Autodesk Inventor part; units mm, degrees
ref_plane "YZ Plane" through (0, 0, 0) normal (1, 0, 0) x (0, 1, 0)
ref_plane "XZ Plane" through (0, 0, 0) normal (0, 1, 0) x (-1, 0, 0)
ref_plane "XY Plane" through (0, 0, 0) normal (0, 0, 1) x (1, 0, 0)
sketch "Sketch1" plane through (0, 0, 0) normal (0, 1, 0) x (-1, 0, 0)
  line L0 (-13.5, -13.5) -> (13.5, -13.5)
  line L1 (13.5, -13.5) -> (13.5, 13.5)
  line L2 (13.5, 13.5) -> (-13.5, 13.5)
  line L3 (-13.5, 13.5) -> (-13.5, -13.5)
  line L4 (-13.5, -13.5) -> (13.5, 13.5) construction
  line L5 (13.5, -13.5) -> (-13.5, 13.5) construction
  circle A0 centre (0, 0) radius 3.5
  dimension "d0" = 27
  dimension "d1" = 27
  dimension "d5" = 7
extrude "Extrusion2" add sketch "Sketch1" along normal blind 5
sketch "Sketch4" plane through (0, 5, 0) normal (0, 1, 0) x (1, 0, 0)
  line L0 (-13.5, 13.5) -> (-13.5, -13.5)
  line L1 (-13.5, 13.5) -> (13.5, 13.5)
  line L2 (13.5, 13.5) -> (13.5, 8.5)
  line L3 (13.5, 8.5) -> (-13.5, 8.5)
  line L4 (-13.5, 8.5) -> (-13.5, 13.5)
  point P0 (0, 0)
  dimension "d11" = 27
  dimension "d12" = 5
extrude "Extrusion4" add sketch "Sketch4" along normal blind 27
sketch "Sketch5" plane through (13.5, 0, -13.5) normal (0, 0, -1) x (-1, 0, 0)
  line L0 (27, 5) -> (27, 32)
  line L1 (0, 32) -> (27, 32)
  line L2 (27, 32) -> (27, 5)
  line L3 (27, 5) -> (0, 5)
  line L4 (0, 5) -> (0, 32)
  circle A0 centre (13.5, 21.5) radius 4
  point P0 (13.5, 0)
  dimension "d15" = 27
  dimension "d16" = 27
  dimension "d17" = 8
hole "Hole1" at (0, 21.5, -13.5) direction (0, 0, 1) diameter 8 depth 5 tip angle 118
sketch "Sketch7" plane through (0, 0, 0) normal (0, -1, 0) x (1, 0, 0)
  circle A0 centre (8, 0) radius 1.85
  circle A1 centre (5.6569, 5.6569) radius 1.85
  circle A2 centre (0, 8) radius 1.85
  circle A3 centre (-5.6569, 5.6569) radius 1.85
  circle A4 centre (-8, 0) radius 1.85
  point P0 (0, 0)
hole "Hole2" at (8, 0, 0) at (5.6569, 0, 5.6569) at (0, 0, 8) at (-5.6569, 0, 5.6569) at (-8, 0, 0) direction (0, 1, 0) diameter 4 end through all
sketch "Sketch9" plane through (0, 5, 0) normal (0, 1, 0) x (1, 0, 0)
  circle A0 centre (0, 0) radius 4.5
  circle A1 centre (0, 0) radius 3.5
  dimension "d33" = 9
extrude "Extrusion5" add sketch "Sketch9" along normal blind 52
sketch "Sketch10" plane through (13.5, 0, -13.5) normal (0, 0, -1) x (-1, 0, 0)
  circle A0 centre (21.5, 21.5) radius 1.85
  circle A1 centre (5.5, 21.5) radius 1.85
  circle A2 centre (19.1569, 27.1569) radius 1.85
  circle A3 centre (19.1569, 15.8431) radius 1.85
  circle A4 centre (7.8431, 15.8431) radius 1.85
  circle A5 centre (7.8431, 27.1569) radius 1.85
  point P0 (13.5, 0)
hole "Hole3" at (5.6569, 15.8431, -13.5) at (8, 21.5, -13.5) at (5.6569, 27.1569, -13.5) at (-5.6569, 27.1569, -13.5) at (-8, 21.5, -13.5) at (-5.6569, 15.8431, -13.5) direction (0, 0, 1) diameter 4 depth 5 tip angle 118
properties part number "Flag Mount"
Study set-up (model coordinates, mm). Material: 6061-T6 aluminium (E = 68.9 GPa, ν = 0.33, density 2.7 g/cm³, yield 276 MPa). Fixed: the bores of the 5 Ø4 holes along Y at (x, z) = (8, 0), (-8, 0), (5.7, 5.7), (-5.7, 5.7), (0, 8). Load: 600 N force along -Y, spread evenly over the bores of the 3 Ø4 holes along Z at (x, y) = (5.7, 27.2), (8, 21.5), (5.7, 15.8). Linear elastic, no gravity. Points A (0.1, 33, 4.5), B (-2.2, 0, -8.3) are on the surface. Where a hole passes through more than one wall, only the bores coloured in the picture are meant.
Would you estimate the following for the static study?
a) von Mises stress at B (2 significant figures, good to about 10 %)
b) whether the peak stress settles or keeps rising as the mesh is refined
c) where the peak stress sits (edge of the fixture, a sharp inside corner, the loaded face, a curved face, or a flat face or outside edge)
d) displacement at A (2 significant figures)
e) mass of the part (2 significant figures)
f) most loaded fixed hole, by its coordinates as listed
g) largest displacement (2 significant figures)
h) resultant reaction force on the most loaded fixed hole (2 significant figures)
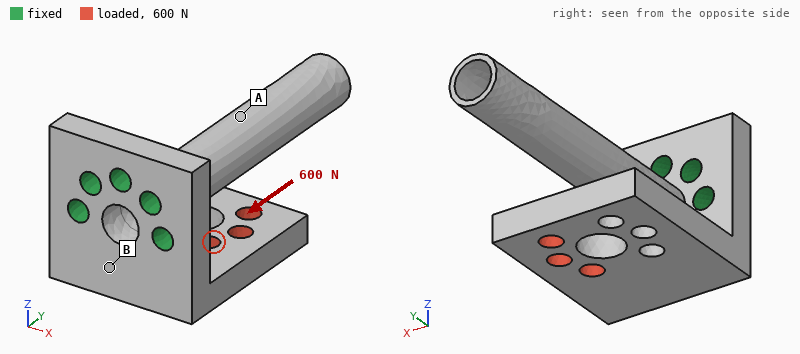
17 MPa
keeps rising
edge of the fixture
11 µm
20 g
(8, 0)
68 µm
570 N
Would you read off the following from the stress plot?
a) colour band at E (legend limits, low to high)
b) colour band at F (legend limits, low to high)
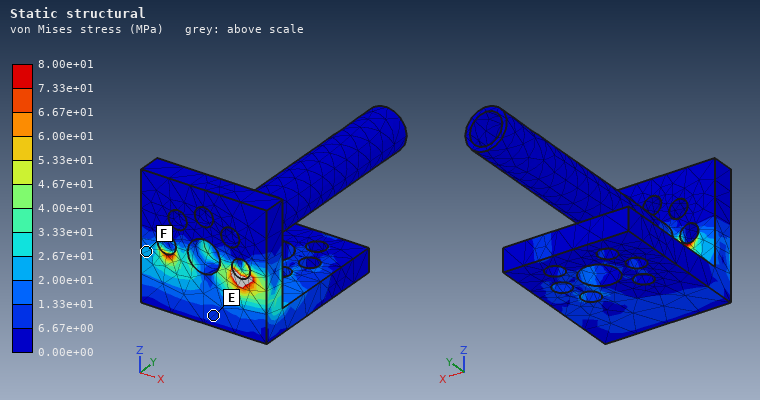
6.67e+00 to 1.33e+01 MPa
2.00e+01 to 2.67e+01 MPa
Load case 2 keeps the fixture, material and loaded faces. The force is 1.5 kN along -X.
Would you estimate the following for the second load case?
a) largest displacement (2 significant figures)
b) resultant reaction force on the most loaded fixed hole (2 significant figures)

0.16 mm
1.9 kN
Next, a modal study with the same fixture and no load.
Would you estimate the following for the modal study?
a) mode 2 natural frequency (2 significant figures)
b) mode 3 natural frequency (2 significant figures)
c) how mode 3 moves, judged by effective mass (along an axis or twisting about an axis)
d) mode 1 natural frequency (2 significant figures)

2700 Hz
3300 Hz
along Z
2600 Hz
